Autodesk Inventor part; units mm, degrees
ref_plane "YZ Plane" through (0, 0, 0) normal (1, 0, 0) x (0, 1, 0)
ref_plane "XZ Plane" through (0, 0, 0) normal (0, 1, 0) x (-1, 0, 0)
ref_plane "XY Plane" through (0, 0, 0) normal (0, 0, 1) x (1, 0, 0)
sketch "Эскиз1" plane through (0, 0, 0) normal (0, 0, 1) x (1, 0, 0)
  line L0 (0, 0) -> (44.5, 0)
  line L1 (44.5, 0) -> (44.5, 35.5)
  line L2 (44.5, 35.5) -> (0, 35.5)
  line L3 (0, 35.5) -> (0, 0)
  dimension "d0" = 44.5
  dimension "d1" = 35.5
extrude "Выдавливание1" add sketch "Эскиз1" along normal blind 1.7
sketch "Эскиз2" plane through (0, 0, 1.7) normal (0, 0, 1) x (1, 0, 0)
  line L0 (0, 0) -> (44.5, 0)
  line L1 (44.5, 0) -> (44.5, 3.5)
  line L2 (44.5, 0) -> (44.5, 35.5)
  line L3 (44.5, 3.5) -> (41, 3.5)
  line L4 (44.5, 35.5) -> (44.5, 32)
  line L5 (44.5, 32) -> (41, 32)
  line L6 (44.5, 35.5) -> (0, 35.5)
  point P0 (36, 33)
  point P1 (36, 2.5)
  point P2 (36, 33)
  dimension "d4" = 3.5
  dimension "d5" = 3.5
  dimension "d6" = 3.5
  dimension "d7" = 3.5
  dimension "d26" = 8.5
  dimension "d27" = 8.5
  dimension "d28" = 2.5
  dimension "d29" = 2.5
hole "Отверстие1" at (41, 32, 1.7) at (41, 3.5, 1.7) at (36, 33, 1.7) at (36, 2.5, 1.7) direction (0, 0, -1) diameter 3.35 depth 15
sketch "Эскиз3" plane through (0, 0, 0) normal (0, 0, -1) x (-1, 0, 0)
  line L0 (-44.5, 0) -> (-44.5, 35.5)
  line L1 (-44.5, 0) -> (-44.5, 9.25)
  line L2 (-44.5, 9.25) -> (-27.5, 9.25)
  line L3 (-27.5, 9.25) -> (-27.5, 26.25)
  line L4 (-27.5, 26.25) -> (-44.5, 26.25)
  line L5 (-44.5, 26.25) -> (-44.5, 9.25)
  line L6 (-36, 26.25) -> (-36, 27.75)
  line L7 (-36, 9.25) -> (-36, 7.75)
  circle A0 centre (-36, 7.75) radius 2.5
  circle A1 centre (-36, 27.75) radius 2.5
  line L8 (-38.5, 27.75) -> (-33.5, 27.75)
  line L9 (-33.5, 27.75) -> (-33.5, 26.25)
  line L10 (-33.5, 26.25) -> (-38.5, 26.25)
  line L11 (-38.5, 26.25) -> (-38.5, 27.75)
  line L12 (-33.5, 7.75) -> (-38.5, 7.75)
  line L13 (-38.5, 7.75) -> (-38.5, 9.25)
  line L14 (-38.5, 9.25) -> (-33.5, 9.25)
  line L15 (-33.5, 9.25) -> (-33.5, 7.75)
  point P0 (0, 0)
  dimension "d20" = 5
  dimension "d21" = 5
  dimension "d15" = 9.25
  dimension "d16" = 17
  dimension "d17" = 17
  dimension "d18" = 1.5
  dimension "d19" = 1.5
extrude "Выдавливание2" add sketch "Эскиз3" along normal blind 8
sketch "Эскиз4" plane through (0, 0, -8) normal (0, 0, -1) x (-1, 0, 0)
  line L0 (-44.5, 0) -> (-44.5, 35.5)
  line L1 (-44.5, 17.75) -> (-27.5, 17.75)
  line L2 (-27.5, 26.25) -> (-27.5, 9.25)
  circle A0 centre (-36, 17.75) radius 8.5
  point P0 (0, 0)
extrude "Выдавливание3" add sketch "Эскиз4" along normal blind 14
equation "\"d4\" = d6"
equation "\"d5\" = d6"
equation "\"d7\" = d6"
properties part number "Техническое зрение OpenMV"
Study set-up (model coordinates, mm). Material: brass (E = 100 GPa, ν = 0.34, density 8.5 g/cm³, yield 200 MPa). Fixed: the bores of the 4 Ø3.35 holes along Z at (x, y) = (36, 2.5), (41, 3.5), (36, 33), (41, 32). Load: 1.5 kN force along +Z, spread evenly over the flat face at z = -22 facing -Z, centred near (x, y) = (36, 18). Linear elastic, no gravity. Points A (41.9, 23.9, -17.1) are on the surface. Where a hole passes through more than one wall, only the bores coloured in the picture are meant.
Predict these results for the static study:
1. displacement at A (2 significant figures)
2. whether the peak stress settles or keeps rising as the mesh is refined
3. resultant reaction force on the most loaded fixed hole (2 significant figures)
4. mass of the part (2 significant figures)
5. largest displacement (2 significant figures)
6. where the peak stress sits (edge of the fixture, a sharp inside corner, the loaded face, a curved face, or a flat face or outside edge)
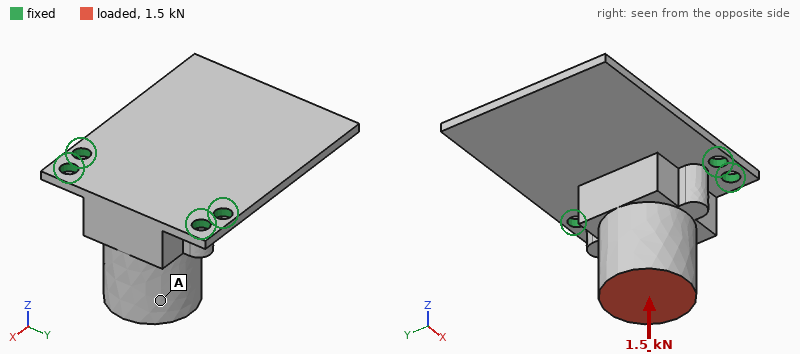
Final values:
23 µm
keeps rising
700 N
71 g
69 µm
edge of the fixture
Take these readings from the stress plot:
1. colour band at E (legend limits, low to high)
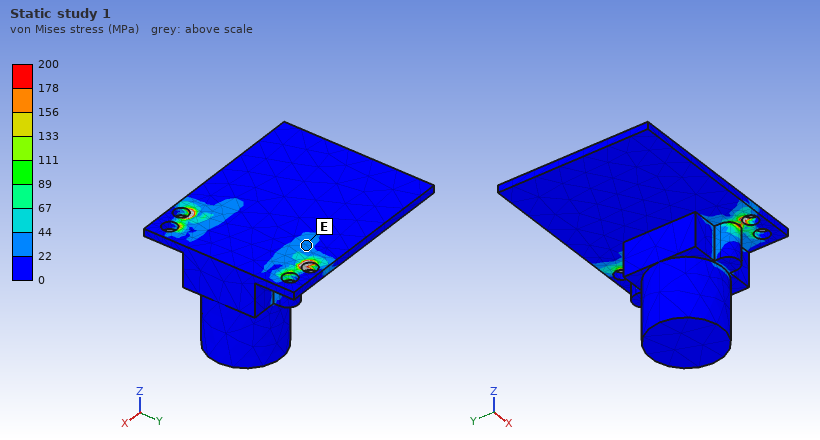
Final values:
22 to 44 MPa
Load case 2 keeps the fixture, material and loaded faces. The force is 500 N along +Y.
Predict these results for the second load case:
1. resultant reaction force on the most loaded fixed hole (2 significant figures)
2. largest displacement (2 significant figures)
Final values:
360 N
15 µm
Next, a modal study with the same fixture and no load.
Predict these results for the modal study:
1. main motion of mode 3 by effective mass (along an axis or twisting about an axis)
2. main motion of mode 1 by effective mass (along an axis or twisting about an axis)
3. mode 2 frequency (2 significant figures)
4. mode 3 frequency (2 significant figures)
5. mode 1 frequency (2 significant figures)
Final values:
along X
along Z
2100 Hz
2300 Hz
980 Hz
